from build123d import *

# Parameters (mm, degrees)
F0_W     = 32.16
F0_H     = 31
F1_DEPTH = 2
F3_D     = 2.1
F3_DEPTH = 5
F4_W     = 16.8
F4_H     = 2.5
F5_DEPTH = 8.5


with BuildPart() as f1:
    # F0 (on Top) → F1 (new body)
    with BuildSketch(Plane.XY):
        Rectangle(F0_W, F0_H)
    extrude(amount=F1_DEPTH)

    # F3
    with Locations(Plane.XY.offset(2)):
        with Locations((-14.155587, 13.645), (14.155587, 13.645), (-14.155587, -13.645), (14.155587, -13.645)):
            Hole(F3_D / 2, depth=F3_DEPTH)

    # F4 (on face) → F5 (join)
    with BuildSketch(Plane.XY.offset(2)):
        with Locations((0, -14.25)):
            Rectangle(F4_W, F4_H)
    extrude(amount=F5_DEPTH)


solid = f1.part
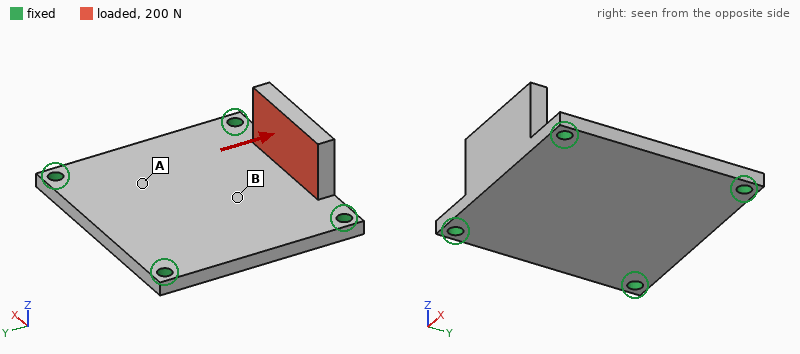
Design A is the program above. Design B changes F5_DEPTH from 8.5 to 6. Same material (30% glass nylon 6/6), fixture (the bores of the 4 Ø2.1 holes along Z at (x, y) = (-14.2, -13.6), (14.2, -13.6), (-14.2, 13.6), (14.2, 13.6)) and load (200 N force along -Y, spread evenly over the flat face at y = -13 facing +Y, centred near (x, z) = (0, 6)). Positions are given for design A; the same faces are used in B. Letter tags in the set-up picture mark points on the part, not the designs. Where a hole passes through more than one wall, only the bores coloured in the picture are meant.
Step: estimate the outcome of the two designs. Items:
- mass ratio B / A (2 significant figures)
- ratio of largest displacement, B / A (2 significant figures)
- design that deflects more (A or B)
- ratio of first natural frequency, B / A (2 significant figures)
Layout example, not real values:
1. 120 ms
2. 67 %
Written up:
1. 0.95
2. 0.56
3. A
4. 1.1
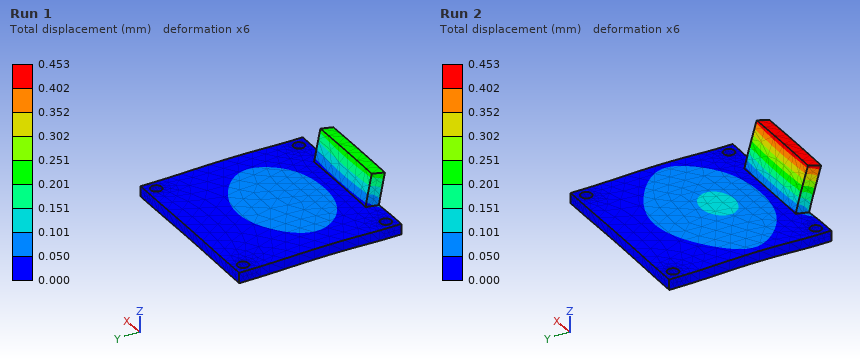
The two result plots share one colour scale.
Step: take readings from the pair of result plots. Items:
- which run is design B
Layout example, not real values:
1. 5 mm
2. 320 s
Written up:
1. Run 1
